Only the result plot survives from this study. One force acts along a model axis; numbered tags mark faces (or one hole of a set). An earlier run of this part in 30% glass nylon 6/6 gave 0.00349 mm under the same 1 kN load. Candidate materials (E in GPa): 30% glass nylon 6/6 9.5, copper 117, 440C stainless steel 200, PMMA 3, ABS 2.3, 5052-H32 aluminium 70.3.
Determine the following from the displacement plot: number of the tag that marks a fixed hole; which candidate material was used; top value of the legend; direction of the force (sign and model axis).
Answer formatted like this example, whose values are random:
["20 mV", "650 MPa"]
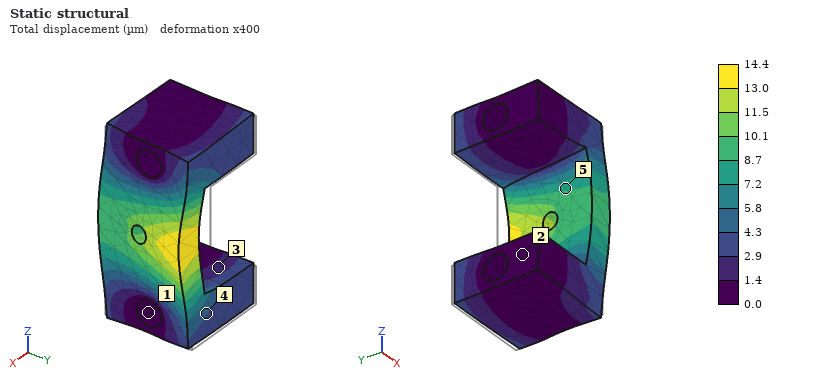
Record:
["1", "ABS", "14.4 µm", "-Y"]
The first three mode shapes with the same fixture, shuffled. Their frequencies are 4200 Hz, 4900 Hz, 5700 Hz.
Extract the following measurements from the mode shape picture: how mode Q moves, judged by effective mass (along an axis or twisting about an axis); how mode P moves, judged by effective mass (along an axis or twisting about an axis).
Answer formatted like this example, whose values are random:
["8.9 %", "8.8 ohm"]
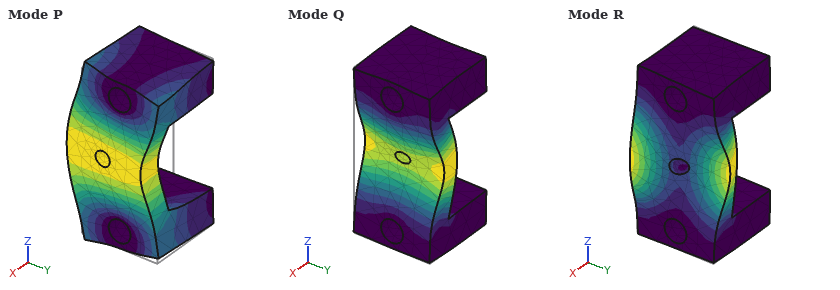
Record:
["along X", "along Y"]
